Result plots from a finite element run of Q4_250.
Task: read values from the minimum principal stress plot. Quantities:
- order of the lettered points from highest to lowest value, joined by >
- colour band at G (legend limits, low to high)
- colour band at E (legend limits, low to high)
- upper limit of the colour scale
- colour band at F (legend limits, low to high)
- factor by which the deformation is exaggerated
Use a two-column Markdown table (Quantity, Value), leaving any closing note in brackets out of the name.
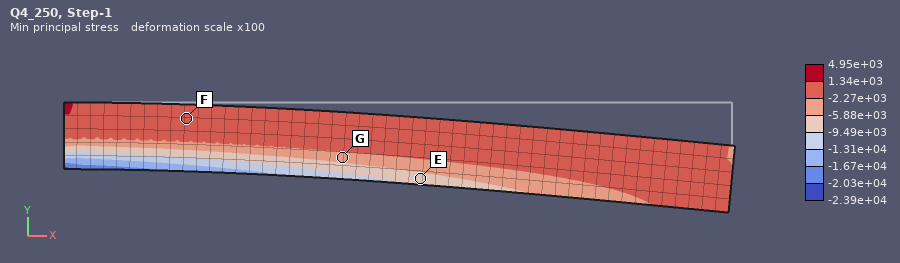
| Quantity | Value |
|---|---|
| order of the lettered points from highest to lowest value, joined by > | F > G > E |
| colour band at G | -5.88e+03 to -2.27e+03 |
| colour band at E | -9.49e+03 to -5.88e+03 |
| upper limit of the colour scale | 4.95e+03 |
| colour band at F | -2.27e+03 to 1.34e+03 |
| factor by which the deformation is exaggerated | 100 |
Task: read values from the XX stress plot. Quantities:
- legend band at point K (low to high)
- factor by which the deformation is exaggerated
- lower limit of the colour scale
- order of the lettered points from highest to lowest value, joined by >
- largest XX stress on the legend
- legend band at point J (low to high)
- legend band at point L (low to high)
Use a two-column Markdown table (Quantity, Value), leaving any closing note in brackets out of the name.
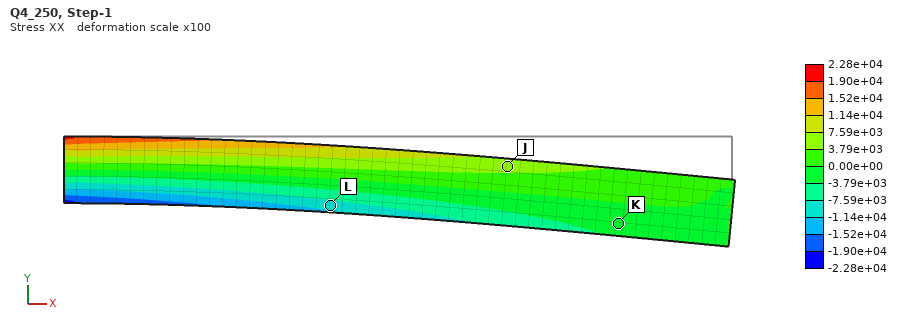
| Quantity | Value |
|---|---|
| legend band at point K | -3.79e+03 to 0.00e+00 |
| factor by which the deformation is exaggerated | 100 |
| lower limit of the colour scale | -2.28e+04 |
| order of the lettered points from highest to lowest value, joined by > | J > K > L |
| largest XX stress on the legend | 2.28e+04 |
| legend band at point J | 3.79e+03 to 7.59e+03 |
| legend band at point L | -1.14e+04 to -7.59e+03 |
